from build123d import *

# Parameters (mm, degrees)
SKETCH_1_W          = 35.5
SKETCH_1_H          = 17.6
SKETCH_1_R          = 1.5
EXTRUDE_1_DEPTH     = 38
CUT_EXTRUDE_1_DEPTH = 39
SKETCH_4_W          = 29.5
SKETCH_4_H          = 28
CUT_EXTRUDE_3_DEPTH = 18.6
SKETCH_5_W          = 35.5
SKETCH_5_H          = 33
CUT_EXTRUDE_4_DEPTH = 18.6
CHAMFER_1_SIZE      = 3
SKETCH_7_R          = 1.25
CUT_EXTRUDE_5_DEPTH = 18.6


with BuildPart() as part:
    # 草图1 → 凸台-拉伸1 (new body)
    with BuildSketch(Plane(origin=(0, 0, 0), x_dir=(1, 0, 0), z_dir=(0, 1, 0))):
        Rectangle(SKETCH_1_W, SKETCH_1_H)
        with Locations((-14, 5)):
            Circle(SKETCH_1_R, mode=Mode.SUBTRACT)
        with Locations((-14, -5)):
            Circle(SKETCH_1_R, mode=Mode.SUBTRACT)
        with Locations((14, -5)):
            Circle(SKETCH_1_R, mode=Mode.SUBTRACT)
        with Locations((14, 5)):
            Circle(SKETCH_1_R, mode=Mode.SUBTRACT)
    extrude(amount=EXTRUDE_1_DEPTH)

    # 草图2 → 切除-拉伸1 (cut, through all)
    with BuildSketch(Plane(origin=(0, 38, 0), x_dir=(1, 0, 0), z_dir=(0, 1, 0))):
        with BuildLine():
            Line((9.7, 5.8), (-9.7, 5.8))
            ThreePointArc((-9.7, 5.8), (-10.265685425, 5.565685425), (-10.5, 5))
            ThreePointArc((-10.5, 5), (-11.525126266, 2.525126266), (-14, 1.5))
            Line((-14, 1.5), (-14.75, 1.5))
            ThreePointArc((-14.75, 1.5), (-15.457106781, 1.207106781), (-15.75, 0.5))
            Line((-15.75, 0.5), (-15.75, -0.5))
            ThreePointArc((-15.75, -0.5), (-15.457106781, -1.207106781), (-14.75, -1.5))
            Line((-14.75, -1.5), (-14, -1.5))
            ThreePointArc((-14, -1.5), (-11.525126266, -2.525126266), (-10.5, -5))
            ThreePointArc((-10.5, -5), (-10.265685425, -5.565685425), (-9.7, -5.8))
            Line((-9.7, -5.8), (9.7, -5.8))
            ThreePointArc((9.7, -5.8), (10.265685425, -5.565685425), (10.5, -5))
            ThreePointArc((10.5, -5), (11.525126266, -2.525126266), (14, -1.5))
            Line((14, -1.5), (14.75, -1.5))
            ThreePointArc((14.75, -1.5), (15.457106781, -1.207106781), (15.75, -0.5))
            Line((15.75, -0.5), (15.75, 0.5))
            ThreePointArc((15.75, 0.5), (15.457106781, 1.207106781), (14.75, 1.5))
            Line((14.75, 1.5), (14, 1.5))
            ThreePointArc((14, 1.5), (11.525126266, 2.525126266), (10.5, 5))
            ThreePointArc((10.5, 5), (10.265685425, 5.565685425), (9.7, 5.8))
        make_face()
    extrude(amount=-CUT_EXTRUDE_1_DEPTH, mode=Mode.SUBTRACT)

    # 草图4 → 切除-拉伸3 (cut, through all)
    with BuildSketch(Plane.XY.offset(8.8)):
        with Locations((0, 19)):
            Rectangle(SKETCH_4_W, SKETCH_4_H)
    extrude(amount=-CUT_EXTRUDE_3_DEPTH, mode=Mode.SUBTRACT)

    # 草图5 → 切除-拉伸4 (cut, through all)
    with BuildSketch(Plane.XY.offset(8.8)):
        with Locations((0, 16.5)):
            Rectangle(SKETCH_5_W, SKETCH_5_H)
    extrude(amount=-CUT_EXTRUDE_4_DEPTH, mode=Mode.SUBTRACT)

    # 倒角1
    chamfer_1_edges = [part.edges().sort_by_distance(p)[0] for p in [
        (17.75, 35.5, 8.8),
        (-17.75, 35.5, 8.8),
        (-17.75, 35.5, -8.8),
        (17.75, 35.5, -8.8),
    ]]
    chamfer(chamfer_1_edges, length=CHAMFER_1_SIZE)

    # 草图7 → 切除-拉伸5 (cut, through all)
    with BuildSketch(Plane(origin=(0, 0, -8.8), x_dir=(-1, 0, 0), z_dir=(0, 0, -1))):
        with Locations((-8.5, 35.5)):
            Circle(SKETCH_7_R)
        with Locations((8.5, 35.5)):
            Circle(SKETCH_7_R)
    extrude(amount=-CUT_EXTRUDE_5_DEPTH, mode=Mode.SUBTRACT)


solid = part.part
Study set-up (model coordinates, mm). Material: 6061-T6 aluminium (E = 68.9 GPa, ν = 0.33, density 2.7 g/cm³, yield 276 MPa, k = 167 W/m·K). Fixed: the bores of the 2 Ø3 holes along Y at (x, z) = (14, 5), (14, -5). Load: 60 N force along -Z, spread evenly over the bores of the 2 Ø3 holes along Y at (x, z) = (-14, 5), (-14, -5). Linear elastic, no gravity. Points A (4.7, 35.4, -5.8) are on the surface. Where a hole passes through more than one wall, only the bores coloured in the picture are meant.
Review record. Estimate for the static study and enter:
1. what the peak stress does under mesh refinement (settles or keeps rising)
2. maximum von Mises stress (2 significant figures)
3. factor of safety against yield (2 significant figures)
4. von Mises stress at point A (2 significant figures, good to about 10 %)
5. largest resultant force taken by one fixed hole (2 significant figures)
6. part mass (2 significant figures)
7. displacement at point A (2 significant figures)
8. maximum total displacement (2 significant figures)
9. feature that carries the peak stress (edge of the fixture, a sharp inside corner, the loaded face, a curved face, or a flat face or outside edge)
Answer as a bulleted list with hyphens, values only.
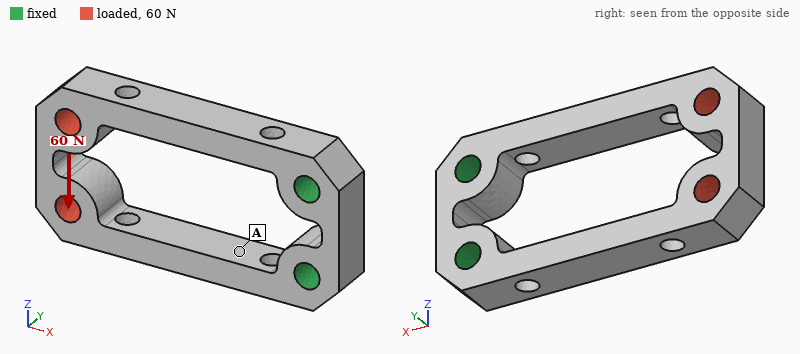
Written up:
- settles
- 120 MPa
- 2.3
- 16 MPa
- 71 N
- 3.8 g
- 16 µm
- 74 µm
- a curved face
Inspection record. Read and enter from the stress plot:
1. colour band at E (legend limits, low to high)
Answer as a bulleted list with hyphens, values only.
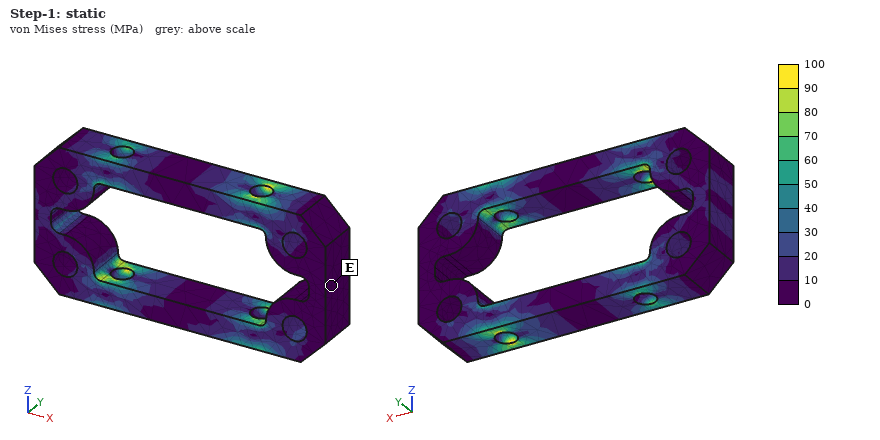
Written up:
- 0 to 10 MPa
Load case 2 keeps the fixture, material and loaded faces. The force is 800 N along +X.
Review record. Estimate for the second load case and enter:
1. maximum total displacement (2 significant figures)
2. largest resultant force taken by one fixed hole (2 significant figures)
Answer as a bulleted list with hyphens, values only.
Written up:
- 38 µm
- 400 N
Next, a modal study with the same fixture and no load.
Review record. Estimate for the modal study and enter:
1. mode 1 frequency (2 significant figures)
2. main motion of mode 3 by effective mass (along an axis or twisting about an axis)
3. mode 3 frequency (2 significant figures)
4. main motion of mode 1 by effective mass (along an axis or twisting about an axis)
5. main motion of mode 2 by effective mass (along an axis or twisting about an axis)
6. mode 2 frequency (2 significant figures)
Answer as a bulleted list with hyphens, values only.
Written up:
- 3300 Hz
- twisting about X
- 7700 Hz
- along Y
- along Z
- 3600 Hz
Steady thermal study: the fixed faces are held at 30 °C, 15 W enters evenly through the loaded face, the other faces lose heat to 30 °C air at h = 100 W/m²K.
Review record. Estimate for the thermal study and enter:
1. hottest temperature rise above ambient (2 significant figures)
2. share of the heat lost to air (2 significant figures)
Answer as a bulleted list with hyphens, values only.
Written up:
- 69 K
- 33 %
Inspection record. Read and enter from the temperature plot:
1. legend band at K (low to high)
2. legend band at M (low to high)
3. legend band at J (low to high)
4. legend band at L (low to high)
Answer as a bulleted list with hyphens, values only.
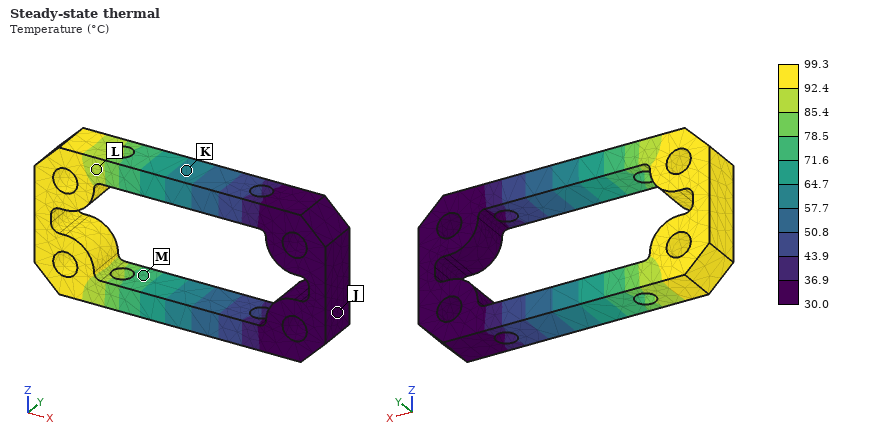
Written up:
- 57.7 to 64.7 °C
- 71.6 to 78.5 °C
- 30.0 to 36.9 °C
- 85.4 to 92.4 °C
